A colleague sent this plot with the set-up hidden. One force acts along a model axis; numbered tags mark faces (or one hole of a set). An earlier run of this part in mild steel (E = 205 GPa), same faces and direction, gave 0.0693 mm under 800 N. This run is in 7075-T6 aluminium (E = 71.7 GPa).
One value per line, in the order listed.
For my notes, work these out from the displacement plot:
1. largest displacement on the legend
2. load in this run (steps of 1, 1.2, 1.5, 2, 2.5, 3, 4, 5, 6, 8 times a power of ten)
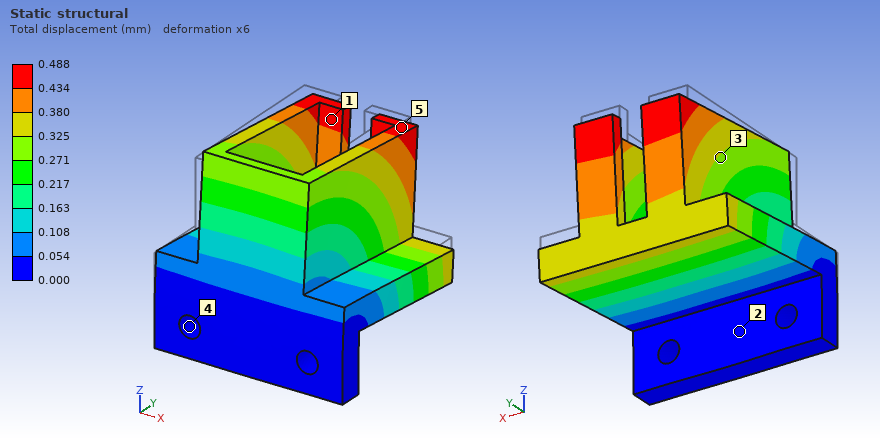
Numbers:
0.488 mm
2 kN
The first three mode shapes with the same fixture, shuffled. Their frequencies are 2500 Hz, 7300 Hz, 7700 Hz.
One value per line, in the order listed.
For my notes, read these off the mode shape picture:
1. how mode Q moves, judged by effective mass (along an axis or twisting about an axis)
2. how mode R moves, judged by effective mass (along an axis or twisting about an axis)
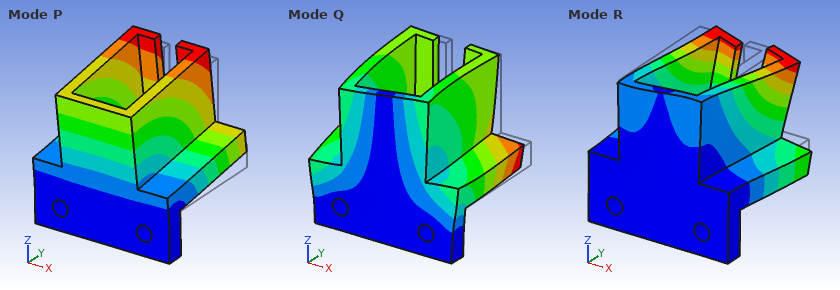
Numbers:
along X
along X
